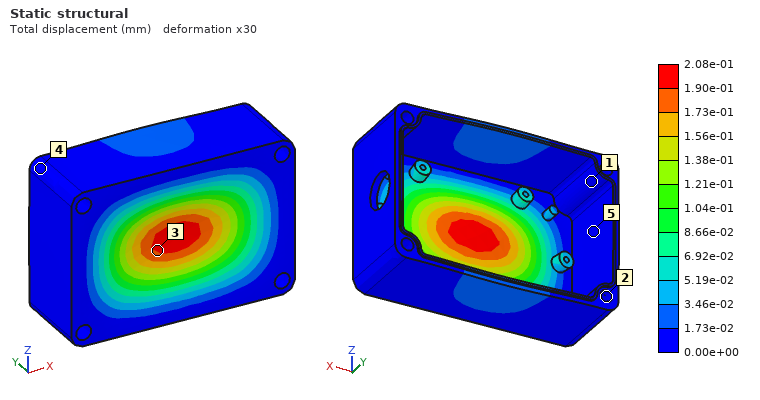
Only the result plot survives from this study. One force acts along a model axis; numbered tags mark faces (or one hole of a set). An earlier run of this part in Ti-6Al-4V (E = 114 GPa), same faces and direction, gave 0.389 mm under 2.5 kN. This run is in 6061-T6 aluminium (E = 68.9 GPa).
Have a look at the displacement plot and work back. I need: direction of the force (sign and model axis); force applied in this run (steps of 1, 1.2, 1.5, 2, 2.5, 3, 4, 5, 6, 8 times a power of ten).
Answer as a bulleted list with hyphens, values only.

- +Y
- 800 N
